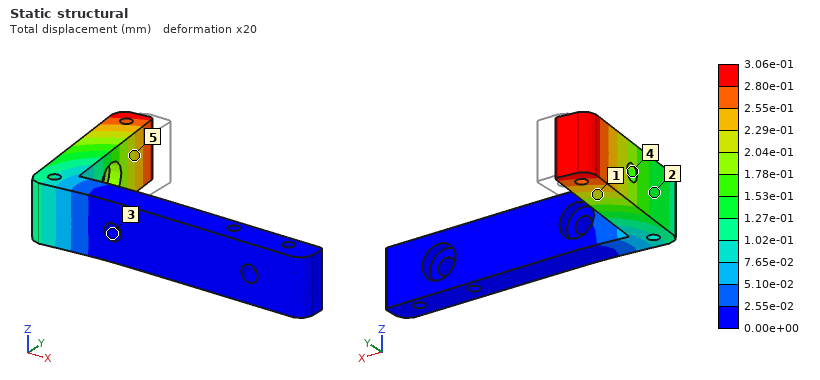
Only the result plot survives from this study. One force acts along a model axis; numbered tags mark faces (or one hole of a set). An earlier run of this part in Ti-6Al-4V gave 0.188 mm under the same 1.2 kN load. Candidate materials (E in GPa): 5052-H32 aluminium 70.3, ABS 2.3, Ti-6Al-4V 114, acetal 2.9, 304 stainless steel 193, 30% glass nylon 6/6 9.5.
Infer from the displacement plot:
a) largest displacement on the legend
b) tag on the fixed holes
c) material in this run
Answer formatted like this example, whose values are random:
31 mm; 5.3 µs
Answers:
3.06e-01 mm; 3; 5052-H32 aluminium
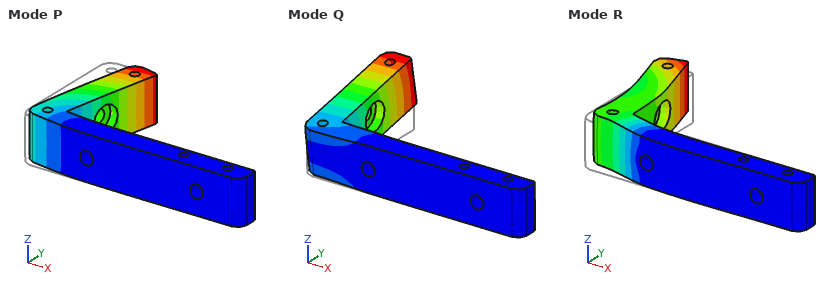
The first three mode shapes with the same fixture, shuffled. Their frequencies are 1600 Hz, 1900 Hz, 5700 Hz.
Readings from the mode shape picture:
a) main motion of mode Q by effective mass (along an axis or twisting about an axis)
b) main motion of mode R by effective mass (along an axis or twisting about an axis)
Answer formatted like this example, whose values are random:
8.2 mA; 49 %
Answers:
along Z; along Y
